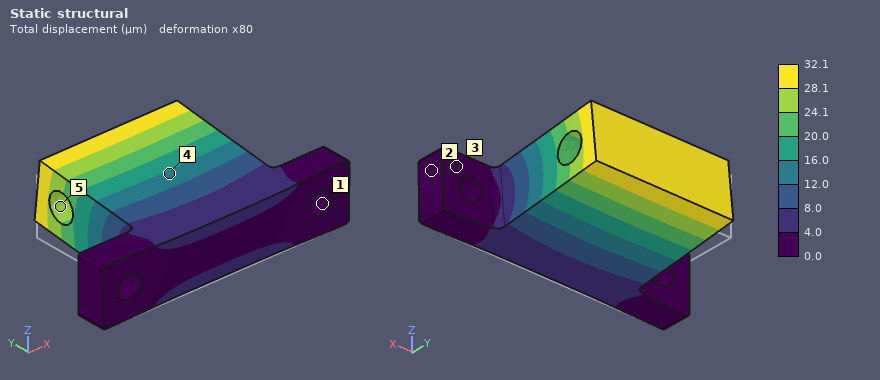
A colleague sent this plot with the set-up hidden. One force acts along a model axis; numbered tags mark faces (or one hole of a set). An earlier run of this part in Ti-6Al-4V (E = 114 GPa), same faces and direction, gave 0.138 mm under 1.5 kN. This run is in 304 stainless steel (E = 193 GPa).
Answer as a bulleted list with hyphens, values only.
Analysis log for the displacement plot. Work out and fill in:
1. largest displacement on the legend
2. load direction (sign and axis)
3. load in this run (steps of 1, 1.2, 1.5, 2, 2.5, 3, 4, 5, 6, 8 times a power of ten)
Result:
- 32.1 µm
- +Z
- 600 N
